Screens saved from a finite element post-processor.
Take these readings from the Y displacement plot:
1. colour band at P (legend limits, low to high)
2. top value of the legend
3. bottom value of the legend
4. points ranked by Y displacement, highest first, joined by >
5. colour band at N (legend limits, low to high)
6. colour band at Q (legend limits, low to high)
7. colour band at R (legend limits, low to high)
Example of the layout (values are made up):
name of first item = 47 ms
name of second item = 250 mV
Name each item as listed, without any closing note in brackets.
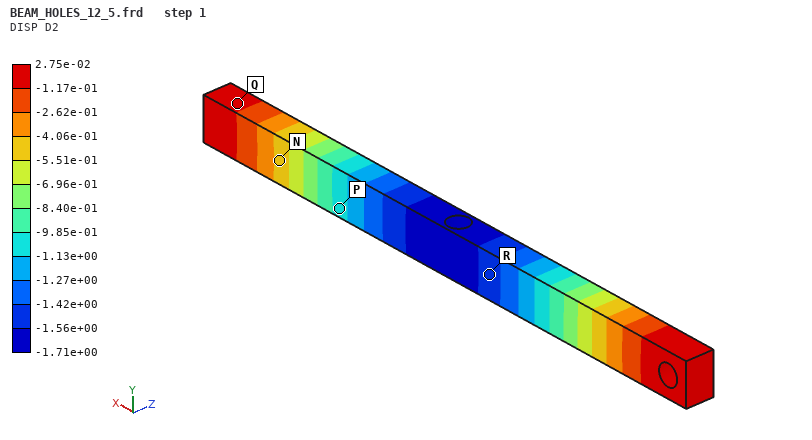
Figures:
colour band at P = -1.13e+00 to -9.85e-01
top value of the legend = 2.75e-02
bottom value of the legend = -1.71e+00
points ranked by Y displacement, highest first, joined by > = Q > N > P > R
colour band at N = -5.51e-01 to -4.06e-01
colour band at Q = -1.17e-01 to 2.75e-02
colour band at R = -1.56e+00 to -1.42e+00
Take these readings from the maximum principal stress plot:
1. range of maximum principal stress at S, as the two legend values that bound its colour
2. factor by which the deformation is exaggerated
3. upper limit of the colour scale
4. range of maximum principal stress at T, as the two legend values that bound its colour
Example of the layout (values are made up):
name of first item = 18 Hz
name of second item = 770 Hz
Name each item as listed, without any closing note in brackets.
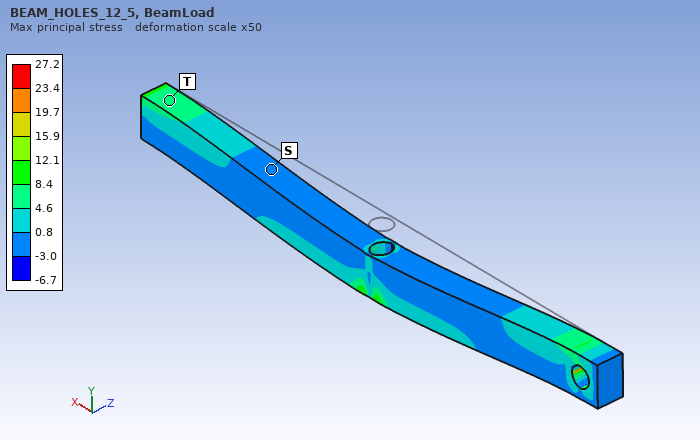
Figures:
range of maximum principal stress at S, as the two legend values that bound its colour = -3.0 to 0.8
factor by which the deformation is exaggerated = 50
upper limit of the colour scale = 27.2
range of maximum principal stress at T, as the two legend values that bound its colour = 4.6 to 8.4
